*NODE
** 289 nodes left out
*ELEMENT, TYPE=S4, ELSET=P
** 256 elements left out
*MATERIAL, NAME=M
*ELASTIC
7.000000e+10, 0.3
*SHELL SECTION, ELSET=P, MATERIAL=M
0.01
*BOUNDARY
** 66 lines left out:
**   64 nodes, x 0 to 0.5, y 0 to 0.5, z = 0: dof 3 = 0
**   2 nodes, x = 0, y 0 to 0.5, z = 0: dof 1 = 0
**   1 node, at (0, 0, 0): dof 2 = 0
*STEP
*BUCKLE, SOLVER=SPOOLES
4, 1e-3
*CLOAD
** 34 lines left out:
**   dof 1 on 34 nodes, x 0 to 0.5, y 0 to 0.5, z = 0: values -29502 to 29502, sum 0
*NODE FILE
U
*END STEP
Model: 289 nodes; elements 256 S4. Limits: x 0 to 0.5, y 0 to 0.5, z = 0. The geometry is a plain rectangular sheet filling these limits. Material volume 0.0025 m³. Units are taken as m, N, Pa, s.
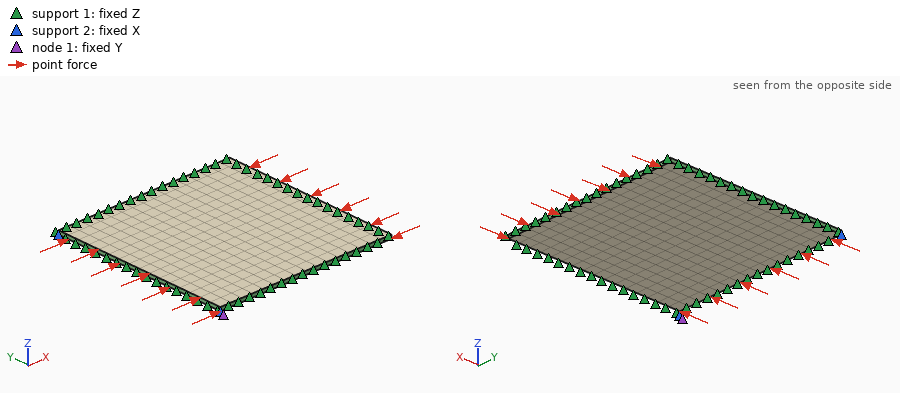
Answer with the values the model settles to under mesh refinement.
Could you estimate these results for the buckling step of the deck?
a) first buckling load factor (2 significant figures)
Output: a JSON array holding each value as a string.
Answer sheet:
["1.1"]
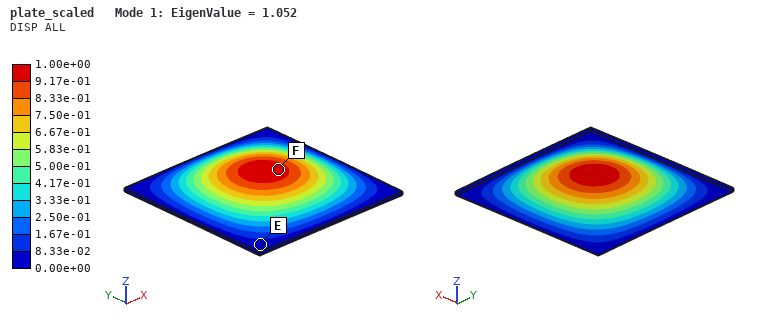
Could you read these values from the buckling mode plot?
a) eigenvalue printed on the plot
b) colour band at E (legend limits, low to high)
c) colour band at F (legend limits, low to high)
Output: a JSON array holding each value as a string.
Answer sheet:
["1.052", "0.00e+00 to 8.33e-02", "9.17e-01 to 1.00e+00"]
